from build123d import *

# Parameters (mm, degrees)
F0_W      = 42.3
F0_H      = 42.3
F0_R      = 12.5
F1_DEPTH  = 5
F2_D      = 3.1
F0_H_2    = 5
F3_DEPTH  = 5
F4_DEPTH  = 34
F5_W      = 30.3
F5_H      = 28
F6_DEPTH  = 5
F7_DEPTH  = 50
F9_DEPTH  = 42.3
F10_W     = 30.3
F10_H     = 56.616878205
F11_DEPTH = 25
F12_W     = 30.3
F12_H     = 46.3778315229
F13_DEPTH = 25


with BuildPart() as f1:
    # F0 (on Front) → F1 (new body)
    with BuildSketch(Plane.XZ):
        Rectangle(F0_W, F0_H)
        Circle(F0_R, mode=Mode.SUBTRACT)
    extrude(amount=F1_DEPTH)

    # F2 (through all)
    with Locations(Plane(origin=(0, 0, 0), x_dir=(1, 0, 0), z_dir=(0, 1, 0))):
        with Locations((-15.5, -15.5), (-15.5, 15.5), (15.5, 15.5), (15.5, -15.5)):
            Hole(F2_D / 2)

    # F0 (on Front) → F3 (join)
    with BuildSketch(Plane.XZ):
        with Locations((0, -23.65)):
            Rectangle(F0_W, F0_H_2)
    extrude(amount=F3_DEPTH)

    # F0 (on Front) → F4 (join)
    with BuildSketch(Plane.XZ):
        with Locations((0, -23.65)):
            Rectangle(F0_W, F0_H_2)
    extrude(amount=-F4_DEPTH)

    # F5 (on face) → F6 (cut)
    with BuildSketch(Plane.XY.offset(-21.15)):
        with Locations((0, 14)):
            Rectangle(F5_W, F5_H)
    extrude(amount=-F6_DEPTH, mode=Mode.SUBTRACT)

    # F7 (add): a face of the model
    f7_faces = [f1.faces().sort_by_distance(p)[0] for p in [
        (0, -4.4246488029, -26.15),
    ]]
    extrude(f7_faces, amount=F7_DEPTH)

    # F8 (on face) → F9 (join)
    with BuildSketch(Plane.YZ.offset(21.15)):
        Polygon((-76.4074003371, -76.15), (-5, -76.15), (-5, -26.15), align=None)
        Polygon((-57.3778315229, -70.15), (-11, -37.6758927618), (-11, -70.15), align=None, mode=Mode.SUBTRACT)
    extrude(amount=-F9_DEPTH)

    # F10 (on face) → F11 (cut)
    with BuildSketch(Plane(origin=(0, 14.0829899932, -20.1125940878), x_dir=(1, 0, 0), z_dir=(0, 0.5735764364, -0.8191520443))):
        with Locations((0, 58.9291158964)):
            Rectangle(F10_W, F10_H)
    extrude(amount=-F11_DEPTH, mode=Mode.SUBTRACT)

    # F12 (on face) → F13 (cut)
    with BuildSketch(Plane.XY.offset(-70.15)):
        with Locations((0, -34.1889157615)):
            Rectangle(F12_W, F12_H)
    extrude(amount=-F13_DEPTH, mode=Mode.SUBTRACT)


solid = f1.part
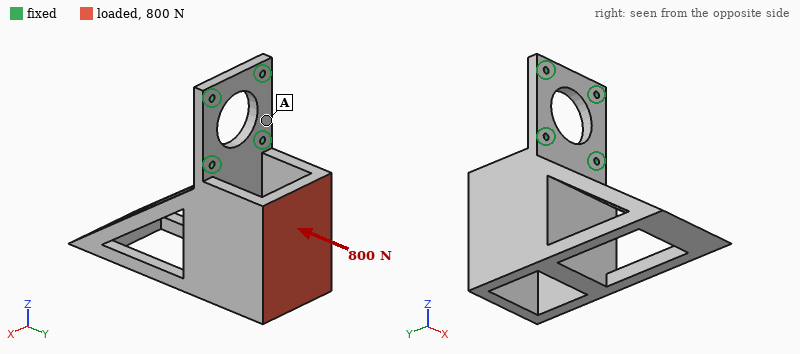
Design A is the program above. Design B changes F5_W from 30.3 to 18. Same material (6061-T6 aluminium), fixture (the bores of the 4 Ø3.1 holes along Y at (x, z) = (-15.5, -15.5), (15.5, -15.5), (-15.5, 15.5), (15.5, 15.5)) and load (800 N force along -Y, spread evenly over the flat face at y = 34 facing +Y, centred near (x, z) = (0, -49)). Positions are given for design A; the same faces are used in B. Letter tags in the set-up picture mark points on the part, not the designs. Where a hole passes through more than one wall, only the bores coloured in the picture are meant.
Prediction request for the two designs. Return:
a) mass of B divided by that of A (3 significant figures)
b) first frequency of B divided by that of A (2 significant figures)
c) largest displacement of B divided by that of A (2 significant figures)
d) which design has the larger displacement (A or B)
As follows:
1.25
0.96
0.92
A
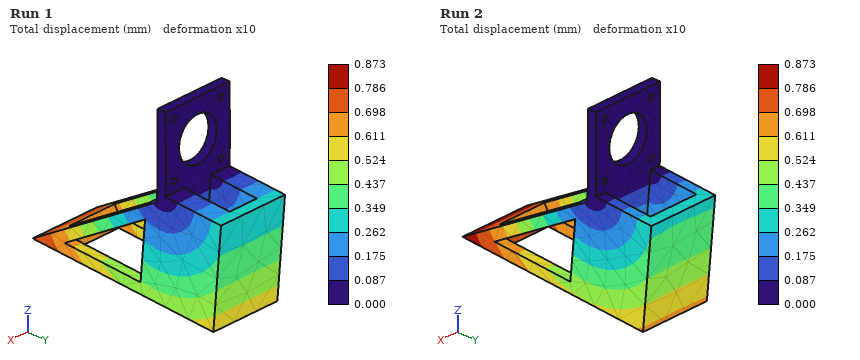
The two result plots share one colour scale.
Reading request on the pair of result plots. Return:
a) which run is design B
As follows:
Run 1
